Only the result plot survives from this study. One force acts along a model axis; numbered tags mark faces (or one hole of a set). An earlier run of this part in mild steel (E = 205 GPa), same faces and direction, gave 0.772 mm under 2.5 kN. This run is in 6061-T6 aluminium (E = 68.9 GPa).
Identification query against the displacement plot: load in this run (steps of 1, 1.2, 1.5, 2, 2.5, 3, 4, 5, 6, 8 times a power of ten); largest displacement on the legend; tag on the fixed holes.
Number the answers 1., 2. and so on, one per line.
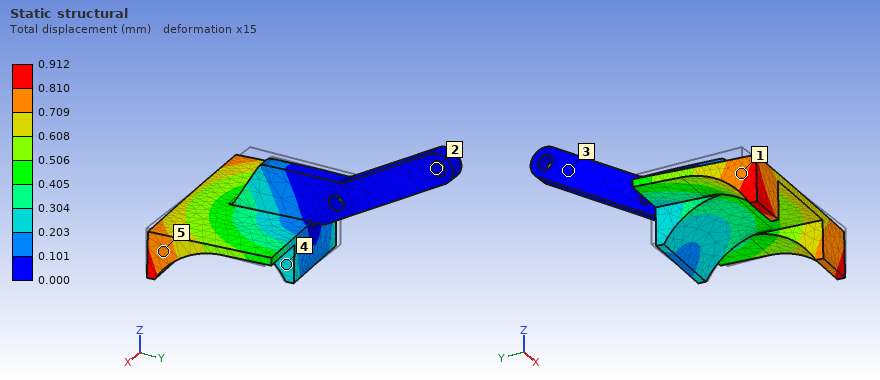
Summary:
1. 1 kN
2. 0.912 mm
3. 2
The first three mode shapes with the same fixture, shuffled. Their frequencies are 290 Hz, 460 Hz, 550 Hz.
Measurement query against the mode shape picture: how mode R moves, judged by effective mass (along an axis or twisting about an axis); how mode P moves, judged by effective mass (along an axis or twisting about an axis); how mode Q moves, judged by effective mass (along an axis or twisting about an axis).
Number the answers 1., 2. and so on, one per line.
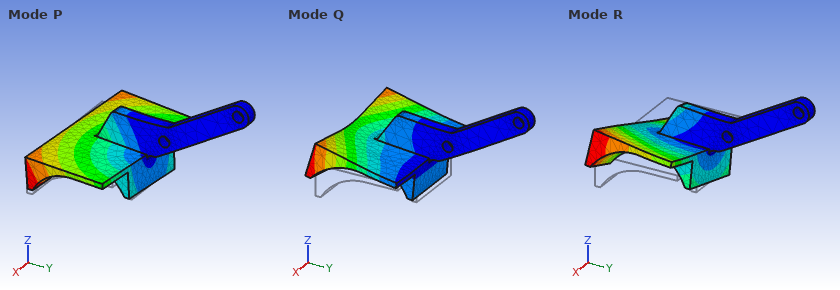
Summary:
1. twisting about Y
2. along X
3. along Z
